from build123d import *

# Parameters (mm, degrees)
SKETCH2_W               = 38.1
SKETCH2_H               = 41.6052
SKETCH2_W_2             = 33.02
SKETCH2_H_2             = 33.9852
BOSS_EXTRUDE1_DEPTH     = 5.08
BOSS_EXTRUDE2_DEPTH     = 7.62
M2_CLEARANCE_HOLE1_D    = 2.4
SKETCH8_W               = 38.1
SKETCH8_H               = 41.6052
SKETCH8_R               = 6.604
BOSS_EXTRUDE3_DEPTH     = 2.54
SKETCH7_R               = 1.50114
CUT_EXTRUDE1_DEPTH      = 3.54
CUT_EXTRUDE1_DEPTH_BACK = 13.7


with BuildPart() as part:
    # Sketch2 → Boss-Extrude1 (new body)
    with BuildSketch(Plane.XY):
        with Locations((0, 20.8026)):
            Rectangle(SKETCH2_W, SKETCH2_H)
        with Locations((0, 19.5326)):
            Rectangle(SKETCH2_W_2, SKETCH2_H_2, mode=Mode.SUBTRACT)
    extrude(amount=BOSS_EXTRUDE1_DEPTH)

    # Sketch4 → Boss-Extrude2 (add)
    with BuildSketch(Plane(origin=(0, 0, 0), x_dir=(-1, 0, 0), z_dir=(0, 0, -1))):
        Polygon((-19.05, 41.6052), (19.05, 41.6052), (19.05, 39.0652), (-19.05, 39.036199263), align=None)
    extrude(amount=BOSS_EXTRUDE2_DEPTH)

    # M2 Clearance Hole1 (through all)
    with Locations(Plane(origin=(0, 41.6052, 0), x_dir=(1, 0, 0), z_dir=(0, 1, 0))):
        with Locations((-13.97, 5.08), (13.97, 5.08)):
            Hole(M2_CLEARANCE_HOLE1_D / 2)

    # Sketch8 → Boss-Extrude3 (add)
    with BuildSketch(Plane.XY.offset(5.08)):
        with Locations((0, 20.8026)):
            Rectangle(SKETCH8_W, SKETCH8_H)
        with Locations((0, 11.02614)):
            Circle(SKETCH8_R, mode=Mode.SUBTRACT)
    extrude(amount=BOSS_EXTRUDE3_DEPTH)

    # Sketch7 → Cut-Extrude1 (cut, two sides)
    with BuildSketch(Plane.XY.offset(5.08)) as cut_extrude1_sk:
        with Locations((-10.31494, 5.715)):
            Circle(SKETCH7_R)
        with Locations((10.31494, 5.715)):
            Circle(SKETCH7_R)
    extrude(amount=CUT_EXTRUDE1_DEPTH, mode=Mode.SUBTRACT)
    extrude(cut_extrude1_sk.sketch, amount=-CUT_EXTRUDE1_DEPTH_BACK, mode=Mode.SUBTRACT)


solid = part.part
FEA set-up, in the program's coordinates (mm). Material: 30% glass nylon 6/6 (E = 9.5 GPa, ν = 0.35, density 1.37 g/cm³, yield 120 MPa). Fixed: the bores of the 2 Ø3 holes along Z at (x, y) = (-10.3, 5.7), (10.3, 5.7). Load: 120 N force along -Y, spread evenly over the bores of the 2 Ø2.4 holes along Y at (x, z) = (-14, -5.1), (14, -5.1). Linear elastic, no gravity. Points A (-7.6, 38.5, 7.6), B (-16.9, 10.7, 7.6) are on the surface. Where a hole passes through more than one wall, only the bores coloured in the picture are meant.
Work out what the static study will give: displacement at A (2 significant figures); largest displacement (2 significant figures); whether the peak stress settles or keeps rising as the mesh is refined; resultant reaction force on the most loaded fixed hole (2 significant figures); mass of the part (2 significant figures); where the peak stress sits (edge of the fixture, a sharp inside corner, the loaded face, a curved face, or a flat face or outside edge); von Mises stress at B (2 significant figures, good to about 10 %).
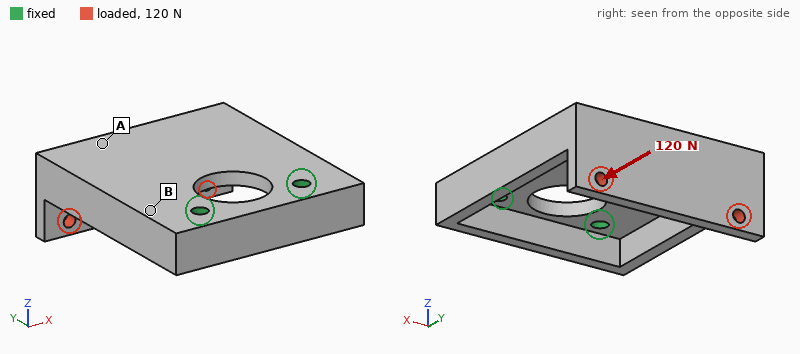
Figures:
0.50 mm
0.68 mm
keeps rising
66 N
9.2 g
edge of the fixture
12 MPa
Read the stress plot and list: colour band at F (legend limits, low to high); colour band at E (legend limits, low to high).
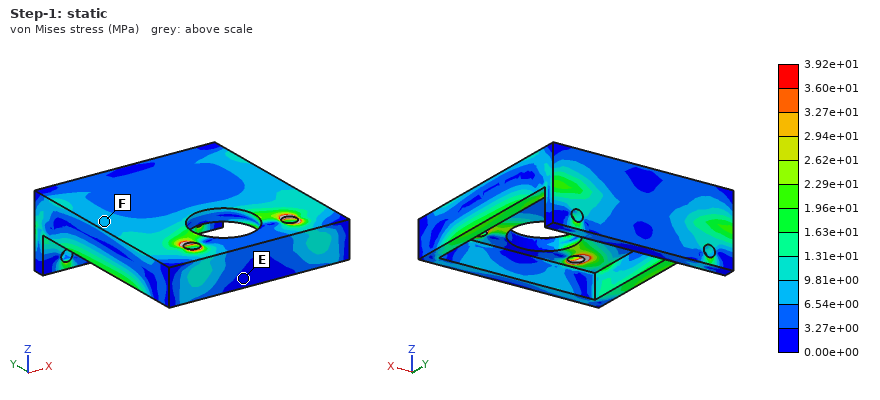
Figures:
6.54e+00 to 9.81e+00 MPa
0.00e+00 to 3.27e+00 MPa
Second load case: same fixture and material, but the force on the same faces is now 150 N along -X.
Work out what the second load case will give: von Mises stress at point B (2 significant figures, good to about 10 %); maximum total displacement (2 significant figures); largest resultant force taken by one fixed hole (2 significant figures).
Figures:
15 MPa
0.66 mm
230 N
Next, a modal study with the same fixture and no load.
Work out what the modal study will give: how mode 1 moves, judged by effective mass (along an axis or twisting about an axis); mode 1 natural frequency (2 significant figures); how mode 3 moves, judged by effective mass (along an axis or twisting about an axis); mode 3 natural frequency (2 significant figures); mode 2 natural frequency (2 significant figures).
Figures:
along Z
720 Hz
along X
3400 Hz
1500 Hz
